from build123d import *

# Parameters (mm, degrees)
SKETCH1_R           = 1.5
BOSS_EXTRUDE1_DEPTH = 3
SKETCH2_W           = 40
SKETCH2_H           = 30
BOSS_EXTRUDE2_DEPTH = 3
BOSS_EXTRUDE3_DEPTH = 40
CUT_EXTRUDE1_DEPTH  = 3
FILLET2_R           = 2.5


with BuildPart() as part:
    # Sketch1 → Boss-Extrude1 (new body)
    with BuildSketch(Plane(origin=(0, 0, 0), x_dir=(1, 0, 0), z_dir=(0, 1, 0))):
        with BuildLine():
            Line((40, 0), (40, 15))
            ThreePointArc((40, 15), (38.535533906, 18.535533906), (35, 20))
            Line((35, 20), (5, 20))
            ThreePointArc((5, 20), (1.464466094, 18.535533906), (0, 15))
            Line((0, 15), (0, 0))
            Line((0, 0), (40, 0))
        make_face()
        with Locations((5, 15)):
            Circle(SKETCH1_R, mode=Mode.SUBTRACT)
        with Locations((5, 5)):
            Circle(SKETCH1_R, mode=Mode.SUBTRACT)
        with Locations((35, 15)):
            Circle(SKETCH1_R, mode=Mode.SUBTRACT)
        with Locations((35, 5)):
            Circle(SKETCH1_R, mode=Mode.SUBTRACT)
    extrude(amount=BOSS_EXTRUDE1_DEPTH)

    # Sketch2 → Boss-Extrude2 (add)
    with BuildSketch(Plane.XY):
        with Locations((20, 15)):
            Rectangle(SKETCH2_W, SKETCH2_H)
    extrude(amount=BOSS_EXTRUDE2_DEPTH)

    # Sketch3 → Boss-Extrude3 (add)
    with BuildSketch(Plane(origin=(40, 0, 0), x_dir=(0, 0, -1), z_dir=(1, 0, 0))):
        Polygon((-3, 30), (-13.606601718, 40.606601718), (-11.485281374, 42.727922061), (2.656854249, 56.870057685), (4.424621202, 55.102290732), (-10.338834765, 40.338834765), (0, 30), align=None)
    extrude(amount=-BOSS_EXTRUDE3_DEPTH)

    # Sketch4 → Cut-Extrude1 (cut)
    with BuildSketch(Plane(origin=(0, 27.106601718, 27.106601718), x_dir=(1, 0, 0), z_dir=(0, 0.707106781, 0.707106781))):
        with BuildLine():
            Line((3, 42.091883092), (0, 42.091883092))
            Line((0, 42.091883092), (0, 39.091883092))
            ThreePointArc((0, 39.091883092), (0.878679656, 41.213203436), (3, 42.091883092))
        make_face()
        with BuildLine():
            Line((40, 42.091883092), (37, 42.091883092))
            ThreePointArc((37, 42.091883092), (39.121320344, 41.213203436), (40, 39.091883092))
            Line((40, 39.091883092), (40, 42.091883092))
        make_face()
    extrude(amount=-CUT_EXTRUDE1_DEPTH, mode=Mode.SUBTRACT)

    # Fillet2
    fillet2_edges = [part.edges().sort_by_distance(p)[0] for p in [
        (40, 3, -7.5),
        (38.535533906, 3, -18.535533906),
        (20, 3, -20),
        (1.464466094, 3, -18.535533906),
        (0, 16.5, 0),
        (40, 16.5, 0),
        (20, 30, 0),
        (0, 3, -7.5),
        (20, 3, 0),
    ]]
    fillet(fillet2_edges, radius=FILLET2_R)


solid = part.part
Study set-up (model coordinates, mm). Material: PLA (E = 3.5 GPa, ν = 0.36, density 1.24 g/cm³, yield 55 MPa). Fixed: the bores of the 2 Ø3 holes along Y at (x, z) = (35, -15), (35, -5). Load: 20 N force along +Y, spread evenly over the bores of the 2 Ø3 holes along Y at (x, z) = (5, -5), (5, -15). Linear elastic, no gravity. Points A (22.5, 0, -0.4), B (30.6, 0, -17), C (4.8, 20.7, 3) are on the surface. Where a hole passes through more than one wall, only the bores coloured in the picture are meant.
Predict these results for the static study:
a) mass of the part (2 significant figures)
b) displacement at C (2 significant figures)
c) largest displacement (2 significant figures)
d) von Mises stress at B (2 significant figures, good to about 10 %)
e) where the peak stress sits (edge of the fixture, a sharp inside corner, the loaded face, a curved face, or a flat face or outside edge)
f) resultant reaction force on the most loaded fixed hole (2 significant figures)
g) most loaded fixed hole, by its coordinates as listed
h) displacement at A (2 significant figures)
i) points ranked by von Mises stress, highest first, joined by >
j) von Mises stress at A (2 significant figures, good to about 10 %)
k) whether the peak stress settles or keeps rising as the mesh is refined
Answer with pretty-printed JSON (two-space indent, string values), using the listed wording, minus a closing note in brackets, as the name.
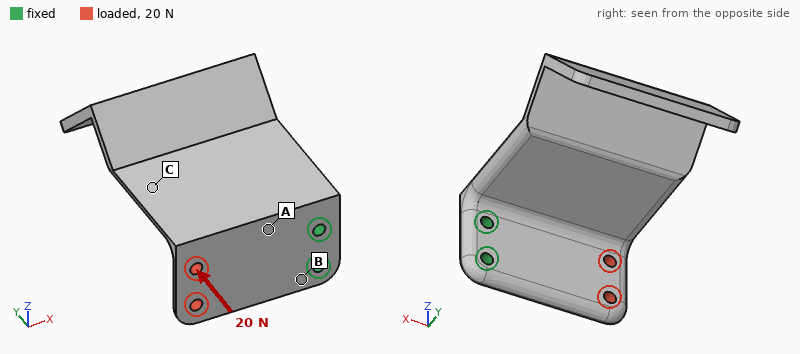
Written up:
{
  "mass of the part": "11 g",
  "displacement at C": "0.43 mm",
  "largest displacement": "0.77 mm",
  "von Mises stress at B": "7.8 MPa",
  "where the peak stress sits": "edge of the fixture",
  "resultant reaction force on the most loaded fixed hole": "12 N",
  "most loaded fixed hole, by its coordinates as listed": "(35, -5)",
  "displacement at A": "0.14 mm",
  "points ranked by von Mises stress, highest first, joined by >": "B > A > C",
  "von Mises stress at A": "2.5 MPa",
  "whether the peak stress settles or keeps rising as the mesh is refined": "keeps rising"
}
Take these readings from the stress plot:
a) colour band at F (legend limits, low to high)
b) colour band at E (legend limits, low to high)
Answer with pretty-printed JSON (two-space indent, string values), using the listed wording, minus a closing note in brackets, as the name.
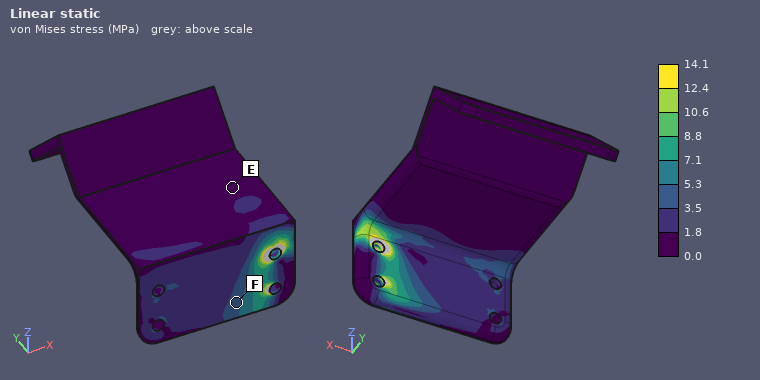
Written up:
{
  "colour band at F": "3.5 to 5.3 MPa",
  "colour band at E": "0.0 to 1.8 MPa"
}
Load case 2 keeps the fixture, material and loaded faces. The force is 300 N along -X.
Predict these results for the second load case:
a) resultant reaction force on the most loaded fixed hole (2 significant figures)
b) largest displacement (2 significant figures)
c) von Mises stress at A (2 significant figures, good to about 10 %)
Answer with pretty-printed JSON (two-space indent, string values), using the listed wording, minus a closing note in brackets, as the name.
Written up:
{
  "resultant reaction force on the most loaded fixed hole": "150 N",
  "largest displacement": "61 µm",
  "von Mises stress at A": "2.2 MPa"
}
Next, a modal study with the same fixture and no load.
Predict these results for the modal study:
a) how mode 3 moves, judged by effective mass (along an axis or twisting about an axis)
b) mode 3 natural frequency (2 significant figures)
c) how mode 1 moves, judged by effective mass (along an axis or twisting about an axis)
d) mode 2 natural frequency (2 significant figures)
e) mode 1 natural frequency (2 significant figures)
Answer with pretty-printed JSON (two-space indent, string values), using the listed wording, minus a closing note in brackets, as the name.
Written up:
{
  "how mode 3 moves, judged by effective mass": "twisting about Y",
  "mode 3 natural frequency": "630 Hz",
  "how mode 1 moves, judged by effective mass": "along Z",
  "mode 2 natural frequency": "290 Hz",
  "mode 1 natural frequency": "190 Hz"
}
